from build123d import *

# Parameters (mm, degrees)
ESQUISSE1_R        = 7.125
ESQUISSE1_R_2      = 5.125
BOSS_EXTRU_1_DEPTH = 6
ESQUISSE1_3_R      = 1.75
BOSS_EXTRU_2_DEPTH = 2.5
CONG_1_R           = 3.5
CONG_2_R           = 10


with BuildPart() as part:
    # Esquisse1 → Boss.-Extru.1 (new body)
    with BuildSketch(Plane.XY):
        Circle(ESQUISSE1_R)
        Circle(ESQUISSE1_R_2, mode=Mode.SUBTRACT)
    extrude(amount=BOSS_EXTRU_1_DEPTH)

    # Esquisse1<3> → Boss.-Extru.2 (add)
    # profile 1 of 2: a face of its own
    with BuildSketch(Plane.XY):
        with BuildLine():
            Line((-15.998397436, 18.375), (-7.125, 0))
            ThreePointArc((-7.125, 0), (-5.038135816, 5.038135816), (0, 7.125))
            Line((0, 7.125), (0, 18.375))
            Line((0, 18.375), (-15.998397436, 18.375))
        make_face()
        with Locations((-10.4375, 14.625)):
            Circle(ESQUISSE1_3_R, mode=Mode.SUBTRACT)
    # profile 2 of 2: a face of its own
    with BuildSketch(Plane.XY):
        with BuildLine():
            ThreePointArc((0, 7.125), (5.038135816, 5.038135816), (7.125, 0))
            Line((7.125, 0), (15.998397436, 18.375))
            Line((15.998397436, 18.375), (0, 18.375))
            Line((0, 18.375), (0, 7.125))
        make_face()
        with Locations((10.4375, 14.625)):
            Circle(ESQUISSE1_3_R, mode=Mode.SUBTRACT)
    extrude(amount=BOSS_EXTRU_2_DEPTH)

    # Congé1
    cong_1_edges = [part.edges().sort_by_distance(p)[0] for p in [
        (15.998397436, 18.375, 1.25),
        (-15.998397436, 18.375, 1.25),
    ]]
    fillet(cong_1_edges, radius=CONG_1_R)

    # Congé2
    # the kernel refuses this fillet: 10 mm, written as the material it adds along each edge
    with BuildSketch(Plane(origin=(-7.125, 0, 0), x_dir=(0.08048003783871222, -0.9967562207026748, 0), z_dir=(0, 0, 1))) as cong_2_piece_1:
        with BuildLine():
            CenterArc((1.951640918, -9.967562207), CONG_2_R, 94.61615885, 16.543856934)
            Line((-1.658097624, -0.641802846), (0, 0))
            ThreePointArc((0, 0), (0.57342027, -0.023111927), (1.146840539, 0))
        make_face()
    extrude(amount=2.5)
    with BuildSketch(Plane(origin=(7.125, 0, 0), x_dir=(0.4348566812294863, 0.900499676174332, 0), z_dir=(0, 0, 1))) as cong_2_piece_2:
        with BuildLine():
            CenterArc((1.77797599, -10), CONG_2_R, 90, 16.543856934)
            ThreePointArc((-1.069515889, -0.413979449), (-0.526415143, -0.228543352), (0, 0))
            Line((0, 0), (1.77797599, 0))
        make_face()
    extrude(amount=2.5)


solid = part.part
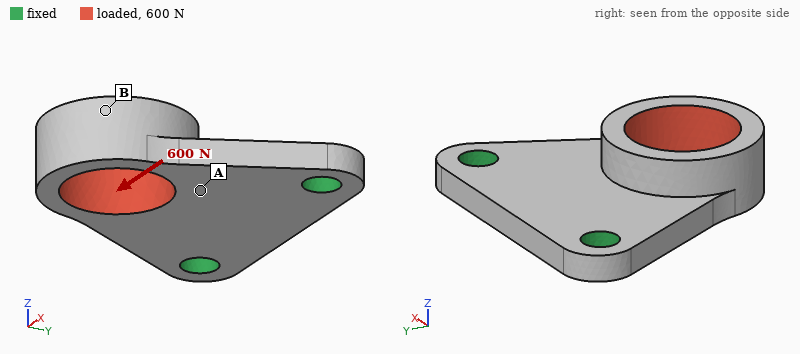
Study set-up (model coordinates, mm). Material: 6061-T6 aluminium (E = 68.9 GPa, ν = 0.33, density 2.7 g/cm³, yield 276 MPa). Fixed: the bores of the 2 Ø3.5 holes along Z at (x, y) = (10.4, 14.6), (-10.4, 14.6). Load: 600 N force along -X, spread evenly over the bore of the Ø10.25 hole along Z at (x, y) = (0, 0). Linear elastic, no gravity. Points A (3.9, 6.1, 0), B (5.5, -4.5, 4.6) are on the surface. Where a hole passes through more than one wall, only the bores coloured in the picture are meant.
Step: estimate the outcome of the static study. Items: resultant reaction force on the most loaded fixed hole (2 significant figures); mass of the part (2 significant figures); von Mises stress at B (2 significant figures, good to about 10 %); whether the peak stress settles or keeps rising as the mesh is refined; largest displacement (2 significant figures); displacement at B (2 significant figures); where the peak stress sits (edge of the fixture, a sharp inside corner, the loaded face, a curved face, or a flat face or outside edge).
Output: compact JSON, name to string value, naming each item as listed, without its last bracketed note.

{"resultant reaction force on the most loaded fixed hole": "500 N", "mass of the part": "3.4 g", "von Mises stress at B": "45 MPa", "whether the peak stress settles or keeps rising as the mesh is refined": "keeps rising", "largest displacement": "38 µm", "displacement at B": "36 µm", "where the peak stress sits": "a sharp inside corner"}
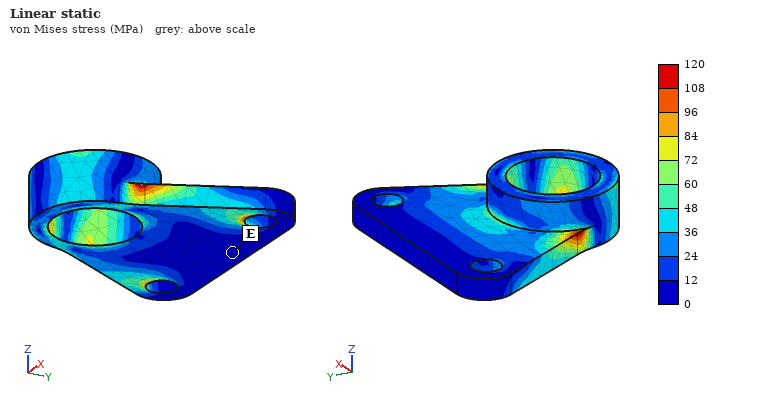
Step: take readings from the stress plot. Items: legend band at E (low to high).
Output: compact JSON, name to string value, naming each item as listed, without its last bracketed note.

{"legend band at E": "0 to 12 MPa"}
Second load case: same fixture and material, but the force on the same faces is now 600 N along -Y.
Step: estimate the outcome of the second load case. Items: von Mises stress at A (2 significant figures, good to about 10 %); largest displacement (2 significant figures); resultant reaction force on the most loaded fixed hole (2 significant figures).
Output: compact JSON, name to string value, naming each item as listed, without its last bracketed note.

{"von Mises stress at A": "37 MPa", "largest displacement": "0.11 mm", "resultant reaction force on the most loaded fixed hole": "320 N"}
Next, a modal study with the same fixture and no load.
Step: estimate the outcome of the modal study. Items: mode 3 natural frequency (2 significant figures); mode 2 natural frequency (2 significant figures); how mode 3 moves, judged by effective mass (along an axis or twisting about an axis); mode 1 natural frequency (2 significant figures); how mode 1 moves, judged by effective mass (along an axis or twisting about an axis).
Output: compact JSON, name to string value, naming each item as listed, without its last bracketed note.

{"mode 3 natural frequency": "22 kHz", "mode 2 natural frequency": "16 kHz", "how mode 3 moves, judged by effective mass": "along X", "mode 1 natural frequency": "5200 Hz", "how mode 1 moves, judged by effective mass": "along Z"}
